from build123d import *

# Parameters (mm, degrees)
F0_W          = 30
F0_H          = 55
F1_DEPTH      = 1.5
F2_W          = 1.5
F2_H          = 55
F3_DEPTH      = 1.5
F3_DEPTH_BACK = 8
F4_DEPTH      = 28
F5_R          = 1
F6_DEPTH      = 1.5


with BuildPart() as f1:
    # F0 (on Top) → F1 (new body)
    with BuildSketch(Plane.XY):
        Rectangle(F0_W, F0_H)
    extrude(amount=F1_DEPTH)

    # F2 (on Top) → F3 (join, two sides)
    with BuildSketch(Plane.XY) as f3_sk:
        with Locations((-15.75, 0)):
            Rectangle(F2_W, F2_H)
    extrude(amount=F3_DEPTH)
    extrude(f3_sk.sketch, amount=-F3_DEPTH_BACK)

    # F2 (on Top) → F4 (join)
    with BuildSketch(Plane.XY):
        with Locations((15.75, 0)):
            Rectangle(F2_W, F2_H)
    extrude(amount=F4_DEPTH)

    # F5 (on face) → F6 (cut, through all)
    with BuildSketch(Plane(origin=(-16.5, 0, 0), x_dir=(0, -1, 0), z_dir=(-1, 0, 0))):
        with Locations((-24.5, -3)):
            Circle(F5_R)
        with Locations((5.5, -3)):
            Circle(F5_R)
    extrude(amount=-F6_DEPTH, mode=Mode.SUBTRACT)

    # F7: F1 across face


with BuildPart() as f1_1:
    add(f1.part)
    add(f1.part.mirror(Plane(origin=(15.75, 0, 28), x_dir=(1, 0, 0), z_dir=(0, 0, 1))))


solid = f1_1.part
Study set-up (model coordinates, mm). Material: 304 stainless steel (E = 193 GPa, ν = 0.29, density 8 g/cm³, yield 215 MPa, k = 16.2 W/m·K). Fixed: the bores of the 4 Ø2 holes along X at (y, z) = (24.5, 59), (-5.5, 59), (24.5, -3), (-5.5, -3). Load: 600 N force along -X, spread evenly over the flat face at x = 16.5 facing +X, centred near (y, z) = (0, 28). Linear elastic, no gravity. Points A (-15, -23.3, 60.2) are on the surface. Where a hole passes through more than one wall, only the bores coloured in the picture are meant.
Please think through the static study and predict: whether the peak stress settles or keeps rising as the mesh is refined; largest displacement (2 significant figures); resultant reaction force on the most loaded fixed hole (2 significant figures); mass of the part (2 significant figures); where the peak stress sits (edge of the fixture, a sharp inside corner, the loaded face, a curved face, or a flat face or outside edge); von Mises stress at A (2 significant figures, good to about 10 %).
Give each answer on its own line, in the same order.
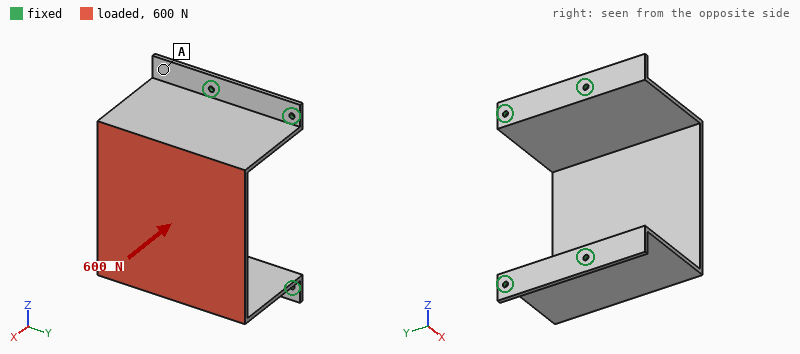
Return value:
keeps rising
0.17 mm
250 N
89 g
edge of the fixture
14 MPa
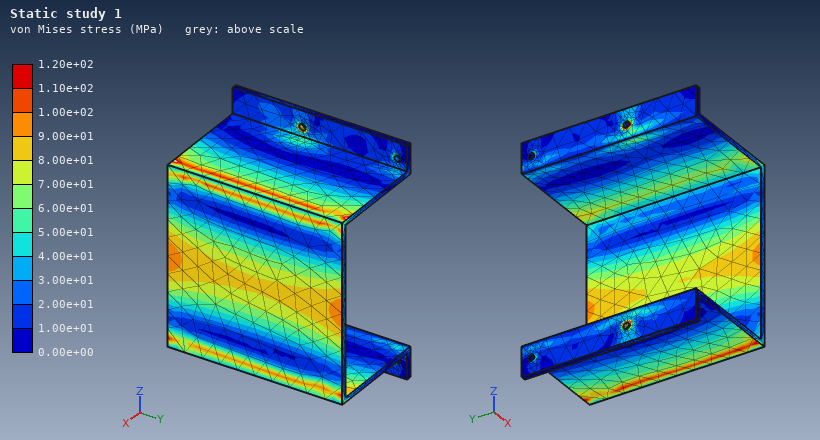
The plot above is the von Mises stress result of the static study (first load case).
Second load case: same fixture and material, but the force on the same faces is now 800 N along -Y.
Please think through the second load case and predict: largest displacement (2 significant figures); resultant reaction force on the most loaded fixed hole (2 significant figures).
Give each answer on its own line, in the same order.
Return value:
43 µm
480 N
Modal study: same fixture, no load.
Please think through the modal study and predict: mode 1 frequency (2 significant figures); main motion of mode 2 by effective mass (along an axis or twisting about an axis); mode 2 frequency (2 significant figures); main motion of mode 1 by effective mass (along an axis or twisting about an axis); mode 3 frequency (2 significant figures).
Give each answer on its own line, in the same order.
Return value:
710 Hz
along X
1900 Hz
along Z
2400 Hz
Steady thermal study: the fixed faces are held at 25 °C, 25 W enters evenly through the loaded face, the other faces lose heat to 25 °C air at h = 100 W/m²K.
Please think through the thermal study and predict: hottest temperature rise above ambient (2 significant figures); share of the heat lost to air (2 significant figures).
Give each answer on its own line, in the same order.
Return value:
64 K
99 %
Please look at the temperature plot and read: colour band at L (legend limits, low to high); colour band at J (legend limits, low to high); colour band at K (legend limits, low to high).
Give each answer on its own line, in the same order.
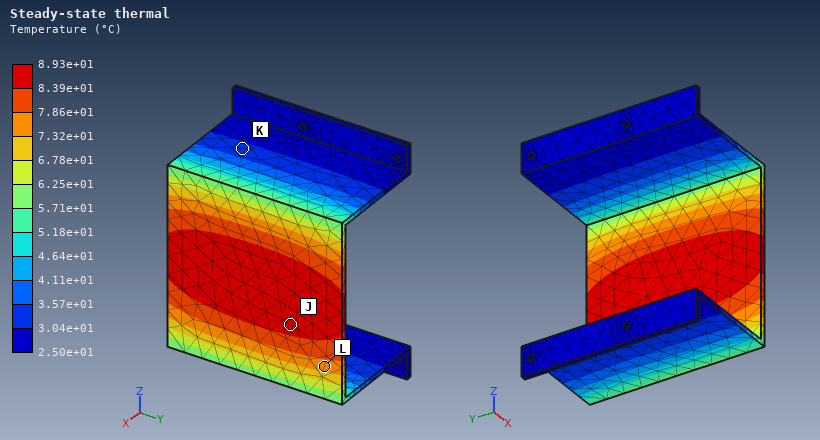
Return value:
7.32e+01 to 7.86e+01 °C
8.39e+01 to 8.93e+01 °C
3.04e+01 to 3.57e+01 °C
